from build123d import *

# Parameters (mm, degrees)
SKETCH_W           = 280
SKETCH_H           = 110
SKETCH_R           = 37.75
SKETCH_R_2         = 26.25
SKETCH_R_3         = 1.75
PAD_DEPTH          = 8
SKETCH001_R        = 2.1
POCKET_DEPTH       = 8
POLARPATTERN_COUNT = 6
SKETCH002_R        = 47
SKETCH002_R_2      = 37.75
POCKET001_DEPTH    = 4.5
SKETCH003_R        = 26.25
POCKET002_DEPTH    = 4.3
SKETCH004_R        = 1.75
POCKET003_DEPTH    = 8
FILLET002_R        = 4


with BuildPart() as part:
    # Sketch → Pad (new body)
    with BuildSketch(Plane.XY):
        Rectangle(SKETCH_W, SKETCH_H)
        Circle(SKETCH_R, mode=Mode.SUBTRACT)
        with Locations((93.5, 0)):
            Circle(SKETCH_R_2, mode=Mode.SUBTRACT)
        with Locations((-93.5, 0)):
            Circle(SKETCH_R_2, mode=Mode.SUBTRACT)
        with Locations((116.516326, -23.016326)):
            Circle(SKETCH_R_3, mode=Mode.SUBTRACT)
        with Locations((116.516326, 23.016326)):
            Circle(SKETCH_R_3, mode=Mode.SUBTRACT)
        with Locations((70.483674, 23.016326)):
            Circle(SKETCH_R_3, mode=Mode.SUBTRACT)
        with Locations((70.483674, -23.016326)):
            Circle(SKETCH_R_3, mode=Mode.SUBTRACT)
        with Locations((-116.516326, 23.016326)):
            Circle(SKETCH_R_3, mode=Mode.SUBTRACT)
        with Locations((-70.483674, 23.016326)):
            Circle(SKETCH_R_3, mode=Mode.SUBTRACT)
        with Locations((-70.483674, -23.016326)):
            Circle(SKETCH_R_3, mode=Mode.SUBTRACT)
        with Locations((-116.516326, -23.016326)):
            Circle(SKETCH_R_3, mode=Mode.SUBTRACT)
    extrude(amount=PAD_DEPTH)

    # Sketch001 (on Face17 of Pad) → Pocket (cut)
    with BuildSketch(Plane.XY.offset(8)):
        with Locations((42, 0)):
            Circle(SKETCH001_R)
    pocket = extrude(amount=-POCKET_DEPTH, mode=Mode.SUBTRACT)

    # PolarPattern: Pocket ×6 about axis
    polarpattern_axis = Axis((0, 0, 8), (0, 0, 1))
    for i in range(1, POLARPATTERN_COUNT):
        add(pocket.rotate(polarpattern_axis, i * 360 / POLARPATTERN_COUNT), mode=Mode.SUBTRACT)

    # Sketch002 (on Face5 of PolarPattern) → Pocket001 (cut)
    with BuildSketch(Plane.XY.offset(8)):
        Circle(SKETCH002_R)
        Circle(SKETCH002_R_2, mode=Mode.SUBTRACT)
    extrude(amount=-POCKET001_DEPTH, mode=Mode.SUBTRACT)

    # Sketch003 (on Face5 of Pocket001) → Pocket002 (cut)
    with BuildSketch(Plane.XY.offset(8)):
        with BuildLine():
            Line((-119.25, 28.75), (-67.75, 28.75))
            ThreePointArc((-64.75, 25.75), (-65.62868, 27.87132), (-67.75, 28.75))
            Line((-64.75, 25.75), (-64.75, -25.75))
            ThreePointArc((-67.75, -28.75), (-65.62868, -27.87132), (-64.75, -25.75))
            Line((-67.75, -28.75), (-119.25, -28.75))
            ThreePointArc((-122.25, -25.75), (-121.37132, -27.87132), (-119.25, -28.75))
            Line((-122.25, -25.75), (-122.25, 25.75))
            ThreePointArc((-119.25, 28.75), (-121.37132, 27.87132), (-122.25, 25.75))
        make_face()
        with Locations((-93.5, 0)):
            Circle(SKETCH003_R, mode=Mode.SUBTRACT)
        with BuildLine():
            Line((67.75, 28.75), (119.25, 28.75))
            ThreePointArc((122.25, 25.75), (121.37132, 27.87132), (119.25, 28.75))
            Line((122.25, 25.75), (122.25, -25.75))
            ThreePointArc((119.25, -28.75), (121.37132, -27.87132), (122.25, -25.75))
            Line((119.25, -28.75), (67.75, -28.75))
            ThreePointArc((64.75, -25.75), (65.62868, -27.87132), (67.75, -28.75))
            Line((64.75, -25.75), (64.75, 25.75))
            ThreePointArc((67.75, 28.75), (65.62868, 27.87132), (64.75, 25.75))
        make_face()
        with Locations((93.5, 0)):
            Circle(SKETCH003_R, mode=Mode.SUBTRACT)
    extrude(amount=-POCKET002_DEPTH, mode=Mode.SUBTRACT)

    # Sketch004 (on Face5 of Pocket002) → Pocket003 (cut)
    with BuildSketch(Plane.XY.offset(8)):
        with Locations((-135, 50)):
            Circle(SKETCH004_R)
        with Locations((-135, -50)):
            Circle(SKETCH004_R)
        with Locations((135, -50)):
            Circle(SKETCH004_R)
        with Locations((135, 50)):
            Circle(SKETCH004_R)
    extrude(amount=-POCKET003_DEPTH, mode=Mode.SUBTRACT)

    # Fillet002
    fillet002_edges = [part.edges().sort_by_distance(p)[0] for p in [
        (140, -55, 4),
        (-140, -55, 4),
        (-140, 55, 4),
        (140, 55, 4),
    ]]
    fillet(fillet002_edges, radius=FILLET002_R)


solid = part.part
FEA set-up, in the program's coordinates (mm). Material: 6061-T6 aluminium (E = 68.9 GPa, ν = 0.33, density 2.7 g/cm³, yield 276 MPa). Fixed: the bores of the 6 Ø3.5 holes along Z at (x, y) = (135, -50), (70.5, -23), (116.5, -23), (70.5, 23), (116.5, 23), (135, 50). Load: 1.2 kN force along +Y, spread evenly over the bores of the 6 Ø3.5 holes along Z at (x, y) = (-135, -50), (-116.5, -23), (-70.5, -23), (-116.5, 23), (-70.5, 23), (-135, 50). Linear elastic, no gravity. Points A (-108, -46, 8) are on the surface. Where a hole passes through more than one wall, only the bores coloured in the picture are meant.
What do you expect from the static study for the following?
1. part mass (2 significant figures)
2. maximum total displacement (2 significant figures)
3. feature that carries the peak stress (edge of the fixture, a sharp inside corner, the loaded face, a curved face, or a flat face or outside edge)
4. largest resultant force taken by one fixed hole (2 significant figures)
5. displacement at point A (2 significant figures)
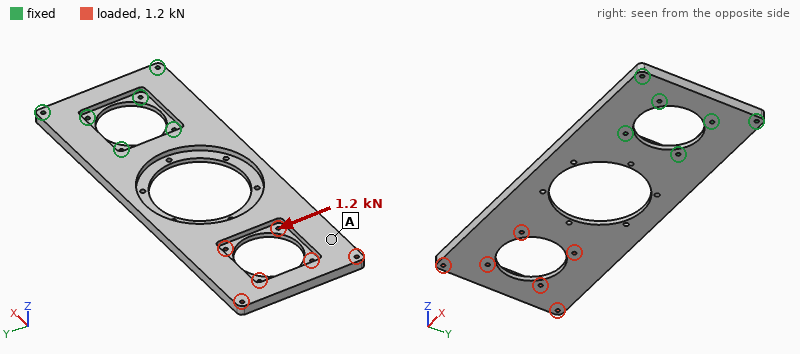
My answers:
420 g
0.27 mm
a curved face
1.5 kN
0.23 mm
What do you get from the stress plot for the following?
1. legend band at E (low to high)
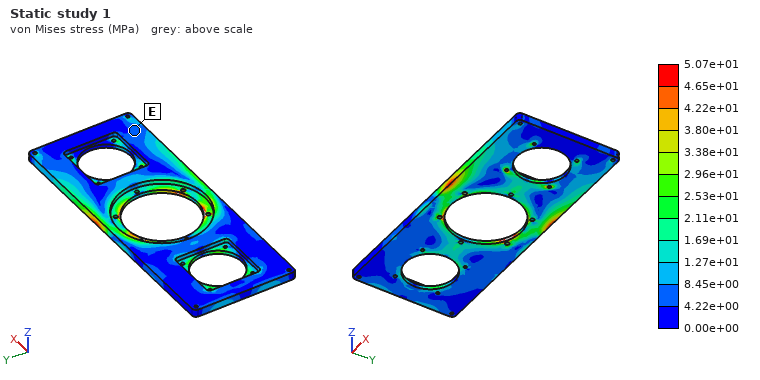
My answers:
4.22e+00 to 8.45e+00 MPa
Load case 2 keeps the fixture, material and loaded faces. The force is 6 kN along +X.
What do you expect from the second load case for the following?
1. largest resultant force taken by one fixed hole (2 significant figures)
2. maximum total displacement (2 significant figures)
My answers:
1.4 kN
0.50 mm
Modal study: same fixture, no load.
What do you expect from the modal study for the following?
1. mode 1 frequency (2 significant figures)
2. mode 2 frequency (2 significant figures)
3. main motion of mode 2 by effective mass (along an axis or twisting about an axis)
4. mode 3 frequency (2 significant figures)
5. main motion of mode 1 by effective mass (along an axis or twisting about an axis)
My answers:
100 Hz
380 Hz
twisting about X
710 Hz
along Z
